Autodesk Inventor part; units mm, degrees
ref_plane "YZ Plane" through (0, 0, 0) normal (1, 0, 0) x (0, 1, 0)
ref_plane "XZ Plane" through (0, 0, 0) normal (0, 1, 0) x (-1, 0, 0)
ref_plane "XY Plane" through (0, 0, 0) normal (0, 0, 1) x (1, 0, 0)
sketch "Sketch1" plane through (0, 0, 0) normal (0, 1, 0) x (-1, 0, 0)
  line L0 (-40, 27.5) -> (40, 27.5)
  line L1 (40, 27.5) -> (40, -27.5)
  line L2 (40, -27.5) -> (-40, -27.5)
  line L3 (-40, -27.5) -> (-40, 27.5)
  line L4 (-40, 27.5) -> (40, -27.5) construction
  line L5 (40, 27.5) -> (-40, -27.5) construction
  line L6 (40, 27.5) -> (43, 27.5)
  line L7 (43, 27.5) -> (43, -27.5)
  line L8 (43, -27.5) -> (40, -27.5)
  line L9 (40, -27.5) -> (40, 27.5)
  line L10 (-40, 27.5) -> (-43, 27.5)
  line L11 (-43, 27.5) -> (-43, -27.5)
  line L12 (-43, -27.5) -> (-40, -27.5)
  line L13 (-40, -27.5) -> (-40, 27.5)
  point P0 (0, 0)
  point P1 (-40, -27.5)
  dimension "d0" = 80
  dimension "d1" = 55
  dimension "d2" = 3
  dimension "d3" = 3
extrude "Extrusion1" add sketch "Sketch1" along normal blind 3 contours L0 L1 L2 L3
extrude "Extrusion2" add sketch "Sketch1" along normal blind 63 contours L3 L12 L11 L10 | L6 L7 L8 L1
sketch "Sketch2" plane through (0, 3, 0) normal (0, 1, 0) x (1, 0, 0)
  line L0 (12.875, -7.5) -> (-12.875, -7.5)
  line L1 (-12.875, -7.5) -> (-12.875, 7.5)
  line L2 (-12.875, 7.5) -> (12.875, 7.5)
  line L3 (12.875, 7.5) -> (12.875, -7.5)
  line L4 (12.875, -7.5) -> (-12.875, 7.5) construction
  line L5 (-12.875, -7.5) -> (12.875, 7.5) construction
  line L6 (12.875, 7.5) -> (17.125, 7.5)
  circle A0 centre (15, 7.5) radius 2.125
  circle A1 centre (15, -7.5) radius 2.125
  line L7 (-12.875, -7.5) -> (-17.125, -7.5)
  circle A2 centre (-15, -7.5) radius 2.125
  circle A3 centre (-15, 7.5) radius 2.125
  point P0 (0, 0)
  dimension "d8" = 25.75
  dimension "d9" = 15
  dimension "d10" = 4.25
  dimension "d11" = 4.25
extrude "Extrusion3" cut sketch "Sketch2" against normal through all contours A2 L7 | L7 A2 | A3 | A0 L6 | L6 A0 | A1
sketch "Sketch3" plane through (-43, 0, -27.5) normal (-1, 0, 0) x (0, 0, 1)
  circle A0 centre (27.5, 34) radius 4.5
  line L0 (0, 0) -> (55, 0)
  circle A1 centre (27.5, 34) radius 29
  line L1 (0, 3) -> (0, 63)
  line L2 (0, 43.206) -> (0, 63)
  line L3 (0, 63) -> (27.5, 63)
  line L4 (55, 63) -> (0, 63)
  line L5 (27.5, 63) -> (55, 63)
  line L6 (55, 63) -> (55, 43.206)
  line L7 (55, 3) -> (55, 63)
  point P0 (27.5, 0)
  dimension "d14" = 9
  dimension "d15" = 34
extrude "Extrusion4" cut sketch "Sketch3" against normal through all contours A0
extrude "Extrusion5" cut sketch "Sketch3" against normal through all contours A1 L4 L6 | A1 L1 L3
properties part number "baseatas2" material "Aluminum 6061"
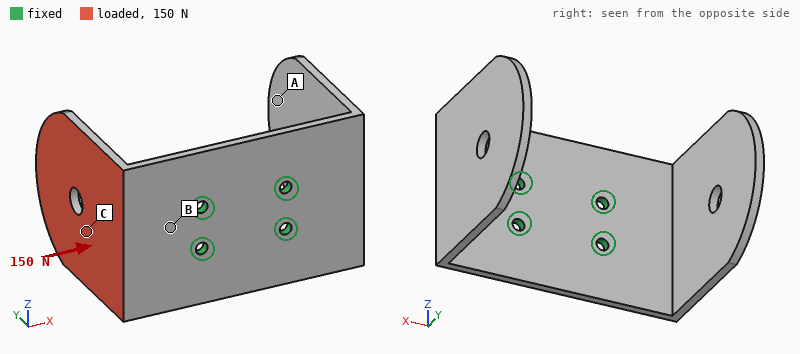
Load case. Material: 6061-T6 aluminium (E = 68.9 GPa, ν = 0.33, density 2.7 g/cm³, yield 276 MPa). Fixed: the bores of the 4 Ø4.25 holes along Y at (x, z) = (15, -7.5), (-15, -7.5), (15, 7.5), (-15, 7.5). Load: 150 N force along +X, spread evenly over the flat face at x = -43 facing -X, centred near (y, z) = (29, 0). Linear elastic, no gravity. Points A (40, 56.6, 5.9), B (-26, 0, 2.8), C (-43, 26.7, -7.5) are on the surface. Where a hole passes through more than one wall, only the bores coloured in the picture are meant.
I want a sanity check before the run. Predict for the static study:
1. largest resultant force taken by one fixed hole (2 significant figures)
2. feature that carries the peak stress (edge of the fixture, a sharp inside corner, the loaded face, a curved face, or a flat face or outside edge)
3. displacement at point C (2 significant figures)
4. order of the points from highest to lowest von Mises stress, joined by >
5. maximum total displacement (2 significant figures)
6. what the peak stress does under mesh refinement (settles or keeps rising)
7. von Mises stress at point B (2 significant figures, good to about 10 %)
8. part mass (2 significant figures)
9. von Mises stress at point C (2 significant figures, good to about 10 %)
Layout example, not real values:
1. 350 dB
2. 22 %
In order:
1. 67 N
2. edge of the fixture
3. 0.45 mm
4. B > C > A
5. 1.2 mm
6. keeps rising
7. 47 MPa
8. 86 g
9. 15 MPa
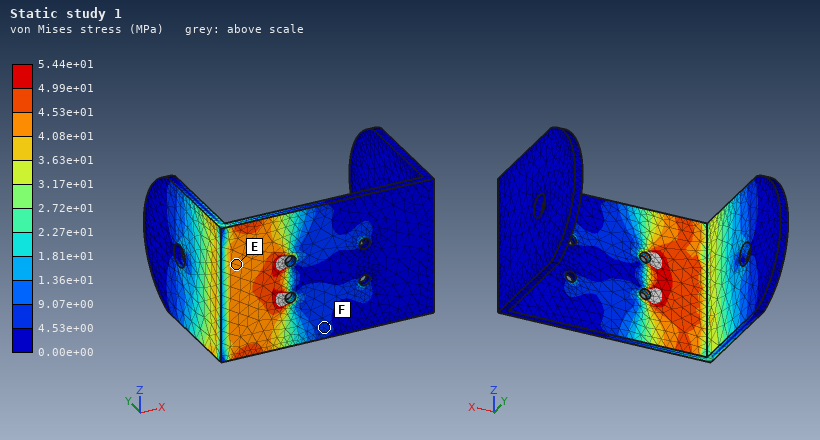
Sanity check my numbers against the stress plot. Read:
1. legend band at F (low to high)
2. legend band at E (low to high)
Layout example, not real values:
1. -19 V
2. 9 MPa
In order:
1. 4.53e+00 to 9.07e+00 MPa
2. 4.08e+01 to 4.53e+01 MPa
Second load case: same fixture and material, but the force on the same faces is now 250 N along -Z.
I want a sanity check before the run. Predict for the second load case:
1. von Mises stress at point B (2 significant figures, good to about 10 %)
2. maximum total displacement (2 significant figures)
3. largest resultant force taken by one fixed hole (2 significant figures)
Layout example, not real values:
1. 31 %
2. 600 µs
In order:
1. 47 MPa
2. 0.50 mm
3. 380 N
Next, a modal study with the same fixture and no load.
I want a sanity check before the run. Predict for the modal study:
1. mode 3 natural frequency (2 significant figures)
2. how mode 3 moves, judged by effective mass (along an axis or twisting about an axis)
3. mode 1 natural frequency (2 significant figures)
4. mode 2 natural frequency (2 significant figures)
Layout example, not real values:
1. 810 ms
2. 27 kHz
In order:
1. 790 Hz
2. twisting about Y
3. 440 Hz
4. 450 Hz
